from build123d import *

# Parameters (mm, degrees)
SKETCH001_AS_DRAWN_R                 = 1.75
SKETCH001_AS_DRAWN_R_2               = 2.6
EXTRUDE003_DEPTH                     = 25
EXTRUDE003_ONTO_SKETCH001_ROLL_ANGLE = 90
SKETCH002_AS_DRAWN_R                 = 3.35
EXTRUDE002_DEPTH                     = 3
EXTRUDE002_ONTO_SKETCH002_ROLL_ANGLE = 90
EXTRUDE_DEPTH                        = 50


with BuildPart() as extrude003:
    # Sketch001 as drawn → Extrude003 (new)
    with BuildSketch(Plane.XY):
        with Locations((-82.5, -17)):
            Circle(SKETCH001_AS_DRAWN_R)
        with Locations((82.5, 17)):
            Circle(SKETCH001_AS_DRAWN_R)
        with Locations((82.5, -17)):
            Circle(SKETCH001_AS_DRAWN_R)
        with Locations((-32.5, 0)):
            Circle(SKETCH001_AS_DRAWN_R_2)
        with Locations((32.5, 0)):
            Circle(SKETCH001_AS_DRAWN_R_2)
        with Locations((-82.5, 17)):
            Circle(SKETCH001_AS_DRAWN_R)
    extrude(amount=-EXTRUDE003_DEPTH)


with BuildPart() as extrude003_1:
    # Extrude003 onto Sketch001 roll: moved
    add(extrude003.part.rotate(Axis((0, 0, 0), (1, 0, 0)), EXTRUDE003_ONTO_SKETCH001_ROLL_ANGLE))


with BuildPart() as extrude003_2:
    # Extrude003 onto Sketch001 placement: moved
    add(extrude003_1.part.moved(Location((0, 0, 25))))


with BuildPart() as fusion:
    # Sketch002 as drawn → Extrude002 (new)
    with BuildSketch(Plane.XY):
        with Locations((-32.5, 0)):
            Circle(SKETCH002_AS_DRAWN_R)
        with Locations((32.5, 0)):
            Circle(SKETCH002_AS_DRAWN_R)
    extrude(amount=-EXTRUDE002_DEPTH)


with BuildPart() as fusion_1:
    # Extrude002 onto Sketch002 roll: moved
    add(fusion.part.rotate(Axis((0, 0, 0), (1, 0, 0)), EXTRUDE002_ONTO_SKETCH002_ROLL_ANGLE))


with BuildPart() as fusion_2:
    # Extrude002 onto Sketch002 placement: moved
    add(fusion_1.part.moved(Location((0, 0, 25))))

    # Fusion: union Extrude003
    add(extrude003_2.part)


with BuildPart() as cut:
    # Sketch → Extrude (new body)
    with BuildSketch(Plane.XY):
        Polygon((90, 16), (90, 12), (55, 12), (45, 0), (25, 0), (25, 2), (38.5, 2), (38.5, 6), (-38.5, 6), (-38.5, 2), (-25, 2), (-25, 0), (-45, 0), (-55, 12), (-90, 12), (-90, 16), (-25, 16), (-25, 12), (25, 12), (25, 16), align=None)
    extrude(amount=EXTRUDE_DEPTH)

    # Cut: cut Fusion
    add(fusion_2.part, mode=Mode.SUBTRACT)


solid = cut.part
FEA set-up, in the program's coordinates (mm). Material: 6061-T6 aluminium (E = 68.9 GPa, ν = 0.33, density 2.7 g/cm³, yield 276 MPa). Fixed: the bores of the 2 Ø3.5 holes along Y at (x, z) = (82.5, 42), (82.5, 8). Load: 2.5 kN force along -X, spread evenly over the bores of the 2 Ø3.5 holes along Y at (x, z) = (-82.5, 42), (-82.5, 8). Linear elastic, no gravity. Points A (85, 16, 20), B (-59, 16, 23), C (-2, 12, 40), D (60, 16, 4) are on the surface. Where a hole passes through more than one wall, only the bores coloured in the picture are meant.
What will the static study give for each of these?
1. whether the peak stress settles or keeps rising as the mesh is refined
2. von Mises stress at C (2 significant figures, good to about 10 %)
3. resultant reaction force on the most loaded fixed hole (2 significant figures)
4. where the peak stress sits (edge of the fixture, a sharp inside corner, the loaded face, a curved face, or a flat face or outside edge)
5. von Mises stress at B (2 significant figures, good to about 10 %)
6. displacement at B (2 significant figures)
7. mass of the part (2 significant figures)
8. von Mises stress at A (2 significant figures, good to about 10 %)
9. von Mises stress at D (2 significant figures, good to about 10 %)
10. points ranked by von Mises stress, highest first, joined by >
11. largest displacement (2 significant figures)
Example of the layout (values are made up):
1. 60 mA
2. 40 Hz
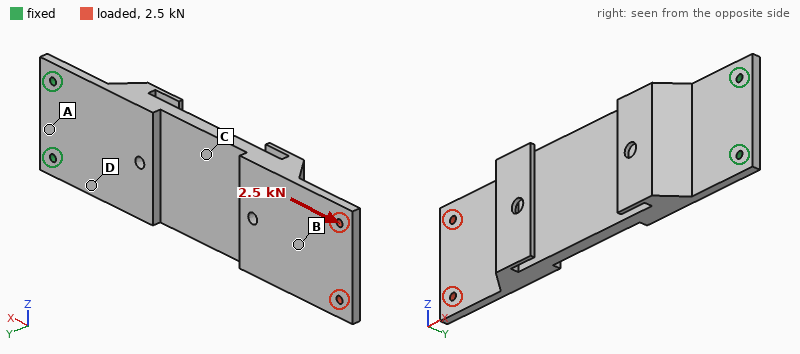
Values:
1. keeps rising
2. 48 MPa
3. 1.3 kN
4. edge of the fixture
5. 11 MPa
6. 0.72 mm
7. 180 g
8. 4.1 MPa
9. 14 MPa
10. C > D > B > A
11. 1.1 mm
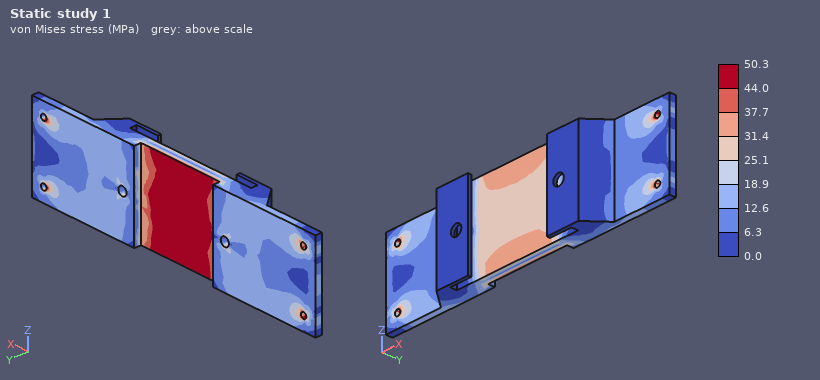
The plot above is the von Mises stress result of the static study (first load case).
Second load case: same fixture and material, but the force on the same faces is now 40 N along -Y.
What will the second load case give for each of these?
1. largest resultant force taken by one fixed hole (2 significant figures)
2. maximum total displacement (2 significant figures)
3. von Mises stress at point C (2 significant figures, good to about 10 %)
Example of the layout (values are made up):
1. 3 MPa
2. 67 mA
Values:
1. 23 N
2. 1.9 mm
3. 10 MPa
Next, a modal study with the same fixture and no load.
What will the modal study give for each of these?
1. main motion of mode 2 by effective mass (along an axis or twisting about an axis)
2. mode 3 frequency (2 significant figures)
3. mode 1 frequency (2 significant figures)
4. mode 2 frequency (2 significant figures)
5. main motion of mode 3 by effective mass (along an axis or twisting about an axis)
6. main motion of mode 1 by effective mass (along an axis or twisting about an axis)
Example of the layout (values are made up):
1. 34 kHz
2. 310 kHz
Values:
1. along Y
2. 1000 Hz
3. 110 Hz
4. 930 Hz
5. along Z
6. along Y
